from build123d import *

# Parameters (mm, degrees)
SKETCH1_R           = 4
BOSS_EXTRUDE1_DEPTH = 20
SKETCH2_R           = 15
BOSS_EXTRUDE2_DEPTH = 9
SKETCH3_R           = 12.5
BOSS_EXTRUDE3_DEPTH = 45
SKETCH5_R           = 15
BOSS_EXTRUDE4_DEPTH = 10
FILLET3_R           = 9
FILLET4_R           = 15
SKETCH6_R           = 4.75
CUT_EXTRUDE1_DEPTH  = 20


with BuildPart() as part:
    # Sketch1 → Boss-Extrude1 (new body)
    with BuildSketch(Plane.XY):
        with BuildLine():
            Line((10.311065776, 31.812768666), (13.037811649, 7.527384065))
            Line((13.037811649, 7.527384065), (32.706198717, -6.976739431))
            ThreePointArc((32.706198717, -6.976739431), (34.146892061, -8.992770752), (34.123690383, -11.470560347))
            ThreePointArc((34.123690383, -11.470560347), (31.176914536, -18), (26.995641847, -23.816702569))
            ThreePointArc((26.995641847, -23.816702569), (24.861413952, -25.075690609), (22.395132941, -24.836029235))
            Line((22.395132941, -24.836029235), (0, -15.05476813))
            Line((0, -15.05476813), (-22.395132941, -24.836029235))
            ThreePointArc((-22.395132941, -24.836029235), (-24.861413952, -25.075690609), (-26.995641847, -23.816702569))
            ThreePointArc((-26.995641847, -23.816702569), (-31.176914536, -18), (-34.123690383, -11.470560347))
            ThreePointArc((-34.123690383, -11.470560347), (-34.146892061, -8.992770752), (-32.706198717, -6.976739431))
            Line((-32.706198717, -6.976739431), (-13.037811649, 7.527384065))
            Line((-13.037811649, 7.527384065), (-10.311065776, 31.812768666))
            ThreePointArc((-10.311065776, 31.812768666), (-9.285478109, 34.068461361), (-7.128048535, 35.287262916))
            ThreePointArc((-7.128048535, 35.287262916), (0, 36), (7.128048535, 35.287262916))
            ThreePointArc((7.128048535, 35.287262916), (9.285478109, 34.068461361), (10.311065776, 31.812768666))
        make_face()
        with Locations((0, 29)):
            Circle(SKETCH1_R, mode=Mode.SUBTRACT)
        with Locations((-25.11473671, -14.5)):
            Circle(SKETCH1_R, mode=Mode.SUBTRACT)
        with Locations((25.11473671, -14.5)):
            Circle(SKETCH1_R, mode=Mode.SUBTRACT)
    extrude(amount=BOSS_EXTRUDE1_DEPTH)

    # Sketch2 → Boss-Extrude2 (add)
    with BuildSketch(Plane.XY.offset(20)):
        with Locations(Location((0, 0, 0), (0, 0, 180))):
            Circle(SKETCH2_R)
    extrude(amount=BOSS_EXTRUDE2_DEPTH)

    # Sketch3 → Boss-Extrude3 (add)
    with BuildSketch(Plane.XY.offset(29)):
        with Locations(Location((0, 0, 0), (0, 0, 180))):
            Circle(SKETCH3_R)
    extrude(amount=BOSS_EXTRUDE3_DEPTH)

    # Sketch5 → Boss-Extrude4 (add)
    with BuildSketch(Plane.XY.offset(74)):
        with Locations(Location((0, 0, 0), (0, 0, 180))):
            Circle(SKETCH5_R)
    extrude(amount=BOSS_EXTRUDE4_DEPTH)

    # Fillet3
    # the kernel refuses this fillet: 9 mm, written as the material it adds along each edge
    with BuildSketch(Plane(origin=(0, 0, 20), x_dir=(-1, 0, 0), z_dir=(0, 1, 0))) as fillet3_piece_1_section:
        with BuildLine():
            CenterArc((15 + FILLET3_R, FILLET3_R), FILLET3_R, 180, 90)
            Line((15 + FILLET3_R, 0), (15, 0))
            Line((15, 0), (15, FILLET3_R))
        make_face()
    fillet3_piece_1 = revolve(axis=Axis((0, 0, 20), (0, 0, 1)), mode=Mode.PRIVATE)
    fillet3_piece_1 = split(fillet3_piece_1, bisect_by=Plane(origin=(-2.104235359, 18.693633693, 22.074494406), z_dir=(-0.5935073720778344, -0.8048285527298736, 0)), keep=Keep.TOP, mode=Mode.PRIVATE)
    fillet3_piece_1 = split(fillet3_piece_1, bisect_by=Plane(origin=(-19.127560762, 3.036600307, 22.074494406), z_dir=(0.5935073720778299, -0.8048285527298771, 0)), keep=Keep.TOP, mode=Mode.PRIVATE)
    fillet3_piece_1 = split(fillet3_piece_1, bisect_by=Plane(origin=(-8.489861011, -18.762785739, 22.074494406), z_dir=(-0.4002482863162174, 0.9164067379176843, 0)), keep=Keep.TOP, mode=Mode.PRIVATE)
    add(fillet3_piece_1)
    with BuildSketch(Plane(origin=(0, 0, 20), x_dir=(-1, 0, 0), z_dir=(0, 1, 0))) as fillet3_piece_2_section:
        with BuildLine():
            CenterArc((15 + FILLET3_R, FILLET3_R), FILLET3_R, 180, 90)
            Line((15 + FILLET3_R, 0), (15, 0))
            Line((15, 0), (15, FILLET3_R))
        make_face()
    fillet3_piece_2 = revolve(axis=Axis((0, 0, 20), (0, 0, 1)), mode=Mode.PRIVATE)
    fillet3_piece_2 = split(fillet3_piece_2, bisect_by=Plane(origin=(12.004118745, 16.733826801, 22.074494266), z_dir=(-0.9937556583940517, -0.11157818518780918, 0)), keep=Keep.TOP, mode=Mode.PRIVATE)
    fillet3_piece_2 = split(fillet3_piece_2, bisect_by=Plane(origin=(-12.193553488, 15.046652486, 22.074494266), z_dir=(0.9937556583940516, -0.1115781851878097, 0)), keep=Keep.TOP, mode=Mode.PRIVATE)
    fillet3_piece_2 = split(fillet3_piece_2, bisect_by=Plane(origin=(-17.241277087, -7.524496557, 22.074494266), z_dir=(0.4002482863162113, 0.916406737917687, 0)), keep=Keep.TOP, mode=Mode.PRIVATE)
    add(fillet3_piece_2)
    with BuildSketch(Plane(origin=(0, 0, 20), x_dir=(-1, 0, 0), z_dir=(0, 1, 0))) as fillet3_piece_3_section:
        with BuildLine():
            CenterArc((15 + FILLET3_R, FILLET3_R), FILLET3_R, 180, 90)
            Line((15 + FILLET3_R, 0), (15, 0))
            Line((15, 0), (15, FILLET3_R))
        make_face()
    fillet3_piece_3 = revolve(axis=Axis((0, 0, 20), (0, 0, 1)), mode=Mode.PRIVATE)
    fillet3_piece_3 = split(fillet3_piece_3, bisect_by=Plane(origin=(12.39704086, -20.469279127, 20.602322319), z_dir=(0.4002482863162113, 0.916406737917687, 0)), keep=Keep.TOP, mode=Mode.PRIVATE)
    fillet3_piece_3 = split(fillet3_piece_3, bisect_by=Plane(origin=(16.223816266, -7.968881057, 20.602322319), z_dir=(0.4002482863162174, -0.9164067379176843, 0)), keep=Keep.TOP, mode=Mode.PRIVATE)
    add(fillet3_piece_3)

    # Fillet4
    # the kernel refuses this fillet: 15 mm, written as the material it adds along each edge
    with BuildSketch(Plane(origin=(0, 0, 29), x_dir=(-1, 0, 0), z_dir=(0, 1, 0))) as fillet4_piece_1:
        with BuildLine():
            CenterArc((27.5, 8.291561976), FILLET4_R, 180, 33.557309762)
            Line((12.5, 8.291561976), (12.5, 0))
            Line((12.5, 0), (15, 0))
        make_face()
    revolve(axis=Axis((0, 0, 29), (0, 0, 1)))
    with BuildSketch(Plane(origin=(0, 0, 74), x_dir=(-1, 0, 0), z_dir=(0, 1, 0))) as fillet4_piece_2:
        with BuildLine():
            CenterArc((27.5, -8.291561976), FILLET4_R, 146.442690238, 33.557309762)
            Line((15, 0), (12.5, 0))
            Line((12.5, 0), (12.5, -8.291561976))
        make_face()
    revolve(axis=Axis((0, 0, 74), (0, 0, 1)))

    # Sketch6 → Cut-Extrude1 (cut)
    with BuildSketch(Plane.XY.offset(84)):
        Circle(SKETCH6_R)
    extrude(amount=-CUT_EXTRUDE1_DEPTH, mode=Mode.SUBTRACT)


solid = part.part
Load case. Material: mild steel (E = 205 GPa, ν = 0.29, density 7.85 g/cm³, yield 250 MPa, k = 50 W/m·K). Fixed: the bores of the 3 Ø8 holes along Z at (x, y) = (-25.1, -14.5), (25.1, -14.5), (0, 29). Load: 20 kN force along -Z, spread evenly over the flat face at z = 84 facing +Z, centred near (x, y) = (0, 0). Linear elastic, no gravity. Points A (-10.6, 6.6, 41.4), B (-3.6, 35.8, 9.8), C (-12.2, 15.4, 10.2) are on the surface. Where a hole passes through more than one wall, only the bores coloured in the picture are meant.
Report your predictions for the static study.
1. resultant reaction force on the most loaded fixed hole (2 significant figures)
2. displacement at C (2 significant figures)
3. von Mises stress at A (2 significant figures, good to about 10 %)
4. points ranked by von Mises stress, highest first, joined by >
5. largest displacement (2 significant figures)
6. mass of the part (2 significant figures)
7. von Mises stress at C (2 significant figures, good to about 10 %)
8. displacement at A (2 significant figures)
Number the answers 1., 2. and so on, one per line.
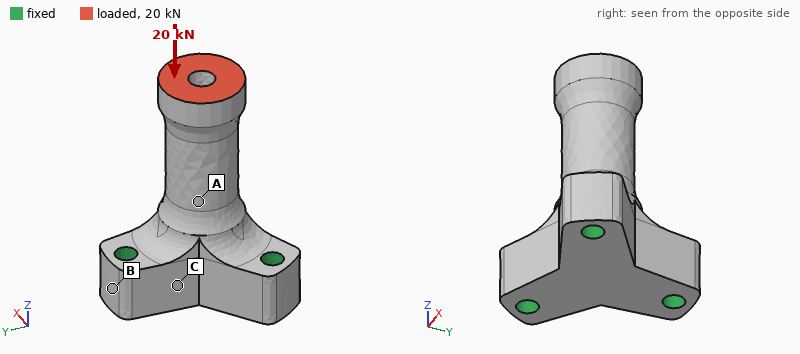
1. 7.0 kN
2. 3.1 µm
3. 42 MPa
4. A > C > B
5. 16 µm
6. 610 g
7. 21 MPa
8. 7.5 µm
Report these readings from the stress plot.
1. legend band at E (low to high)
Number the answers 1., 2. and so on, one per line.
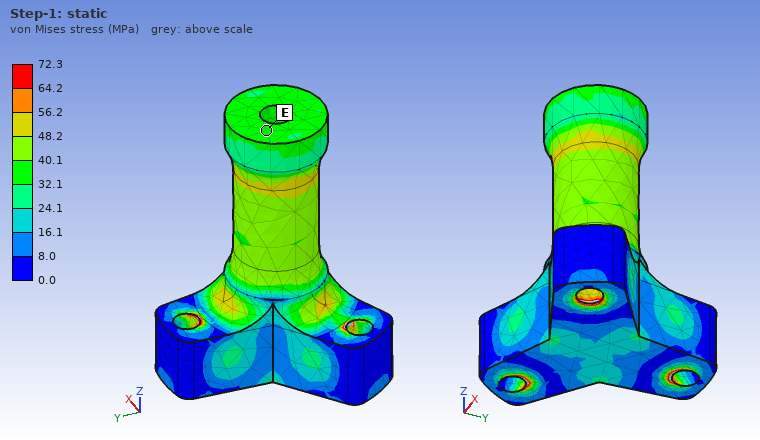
1. 32.1 to 40.1 MPa
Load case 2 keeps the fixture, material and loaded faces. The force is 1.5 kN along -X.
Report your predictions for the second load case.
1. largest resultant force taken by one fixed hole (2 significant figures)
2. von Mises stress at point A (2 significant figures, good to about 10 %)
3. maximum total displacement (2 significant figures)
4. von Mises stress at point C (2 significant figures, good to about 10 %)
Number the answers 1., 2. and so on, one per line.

1. 2.4 kN
2. 37 MPa
3. 35 µm
4. 8.3 MPa
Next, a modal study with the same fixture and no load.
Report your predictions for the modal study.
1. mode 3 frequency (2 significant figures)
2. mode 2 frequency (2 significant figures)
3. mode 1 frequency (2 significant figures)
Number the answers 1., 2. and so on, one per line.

1. 11 kHz
2. 4000 Hz
3. 4000 Hz
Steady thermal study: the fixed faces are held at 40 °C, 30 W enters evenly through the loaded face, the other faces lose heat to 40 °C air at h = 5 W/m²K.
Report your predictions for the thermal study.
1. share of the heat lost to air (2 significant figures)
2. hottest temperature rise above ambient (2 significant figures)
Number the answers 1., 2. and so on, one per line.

1. 5.0 %
2. 79 K
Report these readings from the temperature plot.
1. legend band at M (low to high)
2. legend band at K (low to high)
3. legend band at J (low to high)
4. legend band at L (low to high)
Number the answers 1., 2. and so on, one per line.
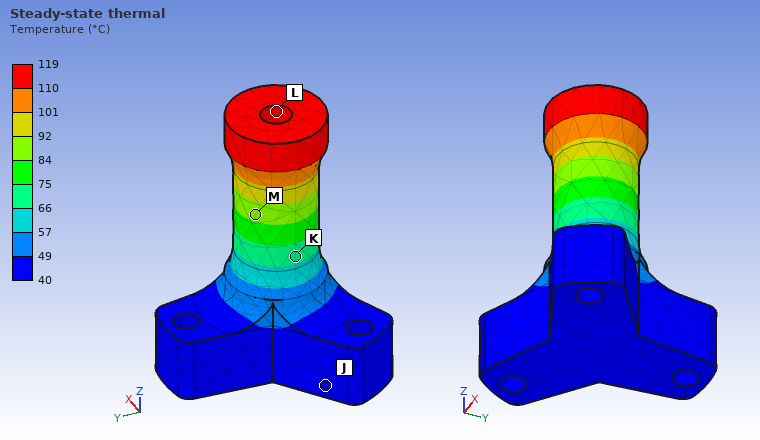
1. 84 to 92 °C
2. 66 to 75 °C
3. 40 to 49 °C
4. 110 to 119 °C
